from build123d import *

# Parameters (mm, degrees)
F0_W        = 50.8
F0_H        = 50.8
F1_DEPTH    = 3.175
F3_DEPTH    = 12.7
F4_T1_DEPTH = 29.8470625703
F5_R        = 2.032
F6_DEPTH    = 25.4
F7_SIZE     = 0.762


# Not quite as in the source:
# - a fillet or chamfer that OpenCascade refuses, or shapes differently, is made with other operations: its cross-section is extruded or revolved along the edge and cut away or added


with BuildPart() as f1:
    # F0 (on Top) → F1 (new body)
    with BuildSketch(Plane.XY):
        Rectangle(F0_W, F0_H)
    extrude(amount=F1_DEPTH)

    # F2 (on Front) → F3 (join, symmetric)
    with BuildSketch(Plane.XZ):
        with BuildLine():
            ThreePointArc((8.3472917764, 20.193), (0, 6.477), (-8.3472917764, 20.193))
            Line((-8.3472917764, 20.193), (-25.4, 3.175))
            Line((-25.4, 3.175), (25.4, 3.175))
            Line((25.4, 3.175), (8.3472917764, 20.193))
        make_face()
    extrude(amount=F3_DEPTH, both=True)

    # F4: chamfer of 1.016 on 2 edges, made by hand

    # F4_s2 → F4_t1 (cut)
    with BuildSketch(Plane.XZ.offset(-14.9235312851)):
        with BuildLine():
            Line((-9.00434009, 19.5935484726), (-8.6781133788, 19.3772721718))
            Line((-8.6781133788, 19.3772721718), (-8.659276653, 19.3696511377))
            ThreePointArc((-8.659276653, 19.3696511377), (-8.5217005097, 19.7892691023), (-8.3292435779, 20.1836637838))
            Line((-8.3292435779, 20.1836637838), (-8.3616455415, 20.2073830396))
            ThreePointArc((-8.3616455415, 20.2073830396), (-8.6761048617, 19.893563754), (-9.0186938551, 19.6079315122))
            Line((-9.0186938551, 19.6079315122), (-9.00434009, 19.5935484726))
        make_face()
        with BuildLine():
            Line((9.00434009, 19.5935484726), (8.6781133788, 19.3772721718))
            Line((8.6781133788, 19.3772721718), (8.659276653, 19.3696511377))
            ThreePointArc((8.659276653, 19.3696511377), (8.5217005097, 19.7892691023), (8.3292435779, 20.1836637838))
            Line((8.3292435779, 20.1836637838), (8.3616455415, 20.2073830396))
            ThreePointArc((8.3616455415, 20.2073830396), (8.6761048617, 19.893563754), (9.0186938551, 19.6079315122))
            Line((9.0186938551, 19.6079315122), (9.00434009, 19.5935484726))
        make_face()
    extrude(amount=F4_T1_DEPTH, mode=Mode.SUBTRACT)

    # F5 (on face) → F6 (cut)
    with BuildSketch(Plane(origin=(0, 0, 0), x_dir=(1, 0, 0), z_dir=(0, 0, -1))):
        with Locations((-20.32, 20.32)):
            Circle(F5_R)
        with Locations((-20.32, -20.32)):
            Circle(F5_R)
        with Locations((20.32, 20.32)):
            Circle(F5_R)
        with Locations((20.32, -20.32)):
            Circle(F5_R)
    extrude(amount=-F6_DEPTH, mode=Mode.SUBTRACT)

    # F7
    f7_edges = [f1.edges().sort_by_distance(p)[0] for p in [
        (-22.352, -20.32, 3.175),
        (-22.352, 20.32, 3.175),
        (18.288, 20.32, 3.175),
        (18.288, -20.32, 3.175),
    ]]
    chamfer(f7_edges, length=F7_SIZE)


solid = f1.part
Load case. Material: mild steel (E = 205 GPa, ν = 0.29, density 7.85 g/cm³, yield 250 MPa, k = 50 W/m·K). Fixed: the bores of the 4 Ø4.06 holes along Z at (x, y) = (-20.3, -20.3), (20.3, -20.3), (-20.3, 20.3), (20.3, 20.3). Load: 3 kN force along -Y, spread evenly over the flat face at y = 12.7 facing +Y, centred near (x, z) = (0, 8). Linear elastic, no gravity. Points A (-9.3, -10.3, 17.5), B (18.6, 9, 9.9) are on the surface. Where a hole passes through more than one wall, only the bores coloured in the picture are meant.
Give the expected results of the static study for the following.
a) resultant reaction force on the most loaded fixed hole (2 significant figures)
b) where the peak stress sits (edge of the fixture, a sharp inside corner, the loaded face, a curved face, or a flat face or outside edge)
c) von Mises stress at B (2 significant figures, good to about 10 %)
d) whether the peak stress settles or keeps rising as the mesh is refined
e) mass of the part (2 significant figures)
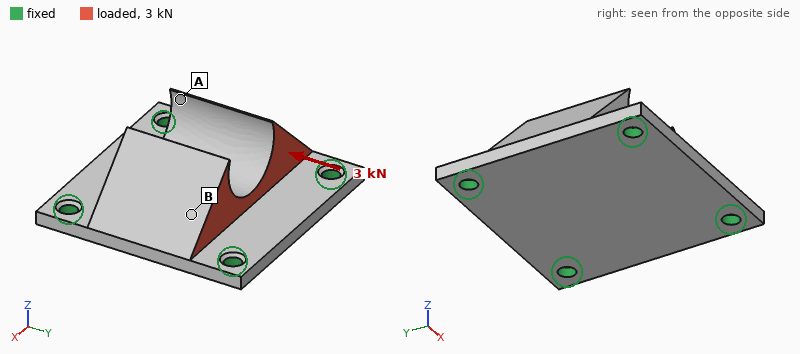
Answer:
860 N
edge of the fixture
10 MPa
keeps rising
130 g
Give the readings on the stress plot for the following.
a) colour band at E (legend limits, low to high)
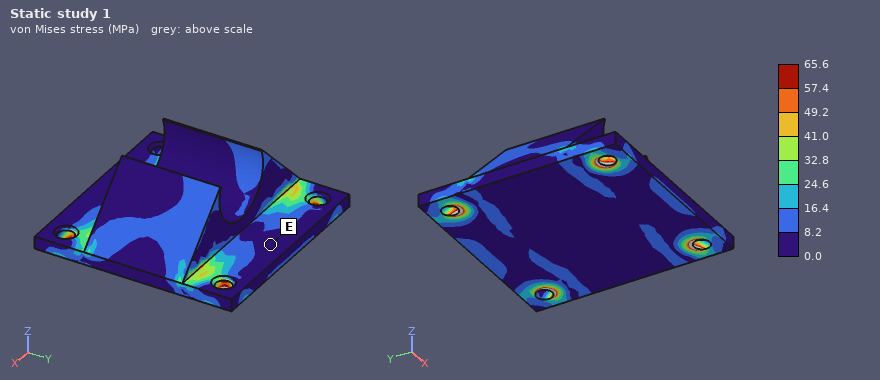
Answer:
0.0 to 8.2 MPa
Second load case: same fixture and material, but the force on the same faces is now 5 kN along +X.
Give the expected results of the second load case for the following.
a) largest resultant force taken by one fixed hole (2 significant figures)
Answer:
1.8 kN
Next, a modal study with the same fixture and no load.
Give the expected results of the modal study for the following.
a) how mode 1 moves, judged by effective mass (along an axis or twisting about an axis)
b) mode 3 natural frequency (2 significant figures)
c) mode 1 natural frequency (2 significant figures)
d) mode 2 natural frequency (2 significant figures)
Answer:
along Z
13 kHz
7400 Hz
11 kHz
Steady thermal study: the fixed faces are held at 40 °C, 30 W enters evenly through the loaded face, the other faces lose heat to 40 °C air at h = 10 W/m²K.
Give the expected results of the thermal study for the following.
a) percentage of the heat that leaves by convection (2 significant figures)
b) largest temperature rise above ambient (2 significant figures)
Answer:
5.2 %
44 K
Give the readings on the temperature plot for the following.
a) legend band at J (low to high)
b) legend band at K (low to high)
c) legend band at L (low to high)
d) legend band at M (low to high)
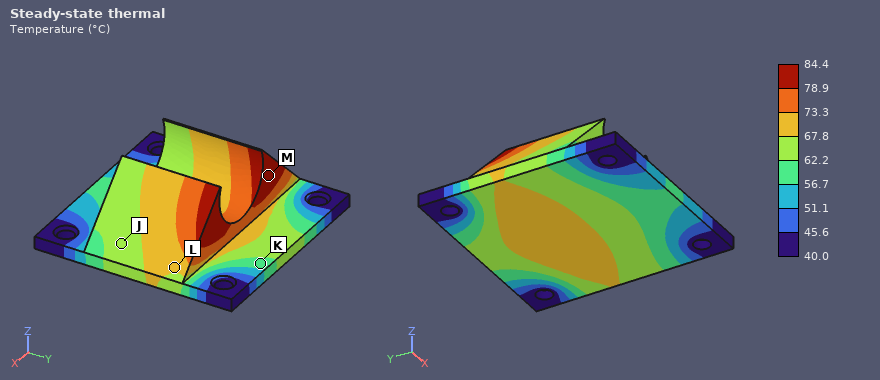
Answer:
62.2 to 67.8 °C
56.7 to 62.2 °C
67.8 to 73.3 °C
78.9 to 84.4 °C
